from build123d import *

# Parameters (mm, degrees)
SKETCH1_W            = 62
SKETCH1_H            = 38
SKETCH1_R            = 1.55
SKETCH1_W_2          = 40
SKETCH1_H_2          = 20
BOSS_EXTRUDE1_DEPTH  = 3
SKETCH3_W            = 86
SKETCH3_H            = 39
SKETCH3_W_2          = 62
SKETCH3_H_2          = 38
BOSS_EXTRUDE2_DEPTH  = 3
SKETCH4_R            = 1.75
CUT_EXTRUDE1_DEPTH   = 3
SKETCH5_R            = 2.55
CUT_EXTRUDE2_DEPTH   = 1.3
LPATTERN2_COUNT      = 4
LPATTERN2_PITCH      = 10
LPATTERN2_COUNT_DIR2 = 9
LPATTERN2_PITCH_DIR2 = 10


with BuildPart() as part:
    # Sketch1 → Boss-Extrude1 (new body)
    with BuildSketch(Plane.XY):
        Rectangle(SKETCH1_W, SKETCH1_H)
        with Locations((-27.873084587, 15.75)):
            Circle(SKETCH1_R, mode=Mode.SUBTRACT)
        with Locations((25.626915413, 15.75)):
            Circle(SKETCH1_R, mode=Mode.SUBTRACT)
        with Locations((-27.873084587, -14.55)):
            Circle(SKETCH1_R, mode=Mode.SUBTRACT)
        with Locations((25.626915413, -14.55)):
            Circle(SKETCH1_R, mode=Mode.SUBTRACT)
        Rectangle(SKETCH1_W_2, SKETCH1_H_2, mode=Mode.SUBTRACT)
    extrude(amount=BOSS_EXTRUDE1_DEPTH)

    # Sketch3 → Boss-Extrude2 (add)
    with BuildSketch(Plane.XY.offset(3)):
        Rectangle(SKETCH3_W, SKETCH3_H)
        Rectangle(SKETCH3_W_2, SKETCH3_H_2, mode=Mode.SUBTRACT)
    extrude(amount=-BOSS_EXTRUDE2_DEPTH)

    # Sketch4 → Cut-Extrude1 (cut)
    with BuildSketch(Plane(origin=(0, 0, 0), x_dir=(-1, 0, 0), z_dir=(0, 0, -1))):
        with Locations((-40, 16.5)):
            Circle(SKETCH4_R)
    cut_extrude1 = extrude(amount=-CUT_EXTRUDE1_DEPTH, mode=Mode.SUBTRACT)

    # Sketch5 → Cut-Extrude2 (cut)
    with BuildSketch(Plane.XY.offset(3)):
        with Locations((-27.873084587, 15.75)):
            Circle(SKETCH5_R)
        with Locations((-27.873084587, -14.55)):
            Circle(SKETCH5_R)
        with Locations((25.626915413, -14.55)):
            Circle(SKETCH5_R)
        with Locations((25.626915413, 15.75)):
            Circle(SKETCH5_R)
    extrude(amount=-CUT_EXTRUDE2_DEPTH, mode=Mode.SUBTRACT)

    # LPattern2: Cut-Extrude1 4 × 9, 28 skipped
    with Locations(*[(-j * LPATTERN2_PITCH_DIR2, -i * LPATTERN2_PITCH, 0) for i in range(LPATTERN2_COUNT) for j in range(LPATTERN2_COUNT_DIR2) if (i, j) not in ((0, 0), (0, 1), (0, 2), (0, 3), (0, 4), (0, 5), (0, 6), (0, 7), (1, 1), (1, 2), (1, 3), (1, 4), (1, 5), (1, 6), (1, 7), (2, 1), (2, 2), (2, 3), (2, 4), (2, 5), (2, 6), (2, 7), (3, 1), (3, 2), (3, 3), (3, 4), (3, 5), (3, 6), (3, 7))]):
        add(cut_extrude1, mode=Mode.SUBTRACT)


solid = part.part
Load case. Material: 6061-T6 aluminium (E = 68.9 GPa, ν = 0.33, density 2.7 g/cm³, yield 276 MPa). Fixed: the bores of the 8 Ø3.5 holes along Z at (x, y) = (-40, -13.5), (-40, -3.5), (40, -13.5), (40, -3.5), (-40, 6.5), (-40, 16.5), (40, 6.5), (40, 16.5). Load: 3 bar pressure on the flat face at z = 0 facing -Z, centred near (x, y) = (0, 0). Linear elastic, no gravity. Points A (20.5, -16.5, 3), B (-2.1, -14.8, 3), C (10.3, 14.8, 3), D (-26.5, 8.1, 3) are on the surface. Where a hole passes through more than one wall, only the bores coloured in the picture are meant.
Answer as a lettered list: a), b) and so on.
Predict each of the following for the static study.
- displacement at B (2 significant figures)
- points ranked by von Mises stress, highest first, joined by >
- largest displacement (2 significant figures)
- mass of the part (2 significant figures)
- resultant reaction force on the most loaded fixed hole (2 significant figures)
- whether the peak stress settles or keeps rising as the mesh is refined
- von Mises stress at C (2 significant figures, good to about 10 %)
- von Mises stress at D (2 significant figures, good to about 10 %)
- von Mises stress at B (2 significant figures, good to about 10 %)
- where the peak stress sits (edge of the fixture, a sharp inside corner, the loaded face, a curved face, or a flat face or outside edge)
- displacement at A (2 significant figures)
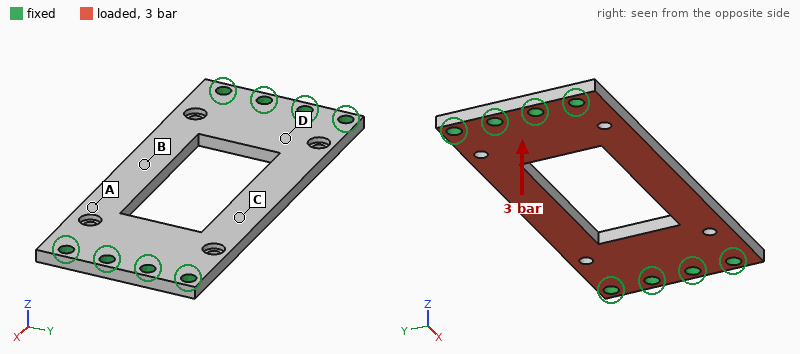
a) 0.15 mm
b) B > C > D > A
c) 0.15 mm
d) 20 g
e) 110 N
f) keeps rising
g) 32 MPa
h) 18 MPa
i) 42 MPa
j) edge of the fixture
k) 0.076 mm
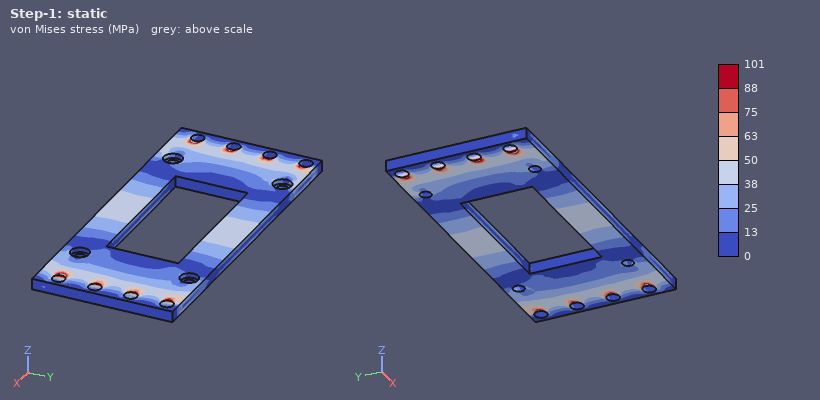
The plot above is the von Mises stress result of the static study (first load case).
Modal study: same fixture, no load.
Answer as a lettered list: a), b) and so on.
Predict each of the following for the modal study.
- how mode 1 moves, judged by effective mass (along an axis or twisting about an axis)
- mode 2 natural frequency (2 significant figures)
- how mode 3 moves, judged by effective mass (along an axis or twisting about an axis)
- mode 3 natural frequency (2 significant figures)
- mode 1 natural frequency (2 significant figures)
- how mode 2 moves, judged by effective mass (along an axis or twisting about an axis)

a) along Z
b) 3500 Hz
c) twisting about Y
d) 7000 Hz
e) 3000 Hz
f) twisting about X
